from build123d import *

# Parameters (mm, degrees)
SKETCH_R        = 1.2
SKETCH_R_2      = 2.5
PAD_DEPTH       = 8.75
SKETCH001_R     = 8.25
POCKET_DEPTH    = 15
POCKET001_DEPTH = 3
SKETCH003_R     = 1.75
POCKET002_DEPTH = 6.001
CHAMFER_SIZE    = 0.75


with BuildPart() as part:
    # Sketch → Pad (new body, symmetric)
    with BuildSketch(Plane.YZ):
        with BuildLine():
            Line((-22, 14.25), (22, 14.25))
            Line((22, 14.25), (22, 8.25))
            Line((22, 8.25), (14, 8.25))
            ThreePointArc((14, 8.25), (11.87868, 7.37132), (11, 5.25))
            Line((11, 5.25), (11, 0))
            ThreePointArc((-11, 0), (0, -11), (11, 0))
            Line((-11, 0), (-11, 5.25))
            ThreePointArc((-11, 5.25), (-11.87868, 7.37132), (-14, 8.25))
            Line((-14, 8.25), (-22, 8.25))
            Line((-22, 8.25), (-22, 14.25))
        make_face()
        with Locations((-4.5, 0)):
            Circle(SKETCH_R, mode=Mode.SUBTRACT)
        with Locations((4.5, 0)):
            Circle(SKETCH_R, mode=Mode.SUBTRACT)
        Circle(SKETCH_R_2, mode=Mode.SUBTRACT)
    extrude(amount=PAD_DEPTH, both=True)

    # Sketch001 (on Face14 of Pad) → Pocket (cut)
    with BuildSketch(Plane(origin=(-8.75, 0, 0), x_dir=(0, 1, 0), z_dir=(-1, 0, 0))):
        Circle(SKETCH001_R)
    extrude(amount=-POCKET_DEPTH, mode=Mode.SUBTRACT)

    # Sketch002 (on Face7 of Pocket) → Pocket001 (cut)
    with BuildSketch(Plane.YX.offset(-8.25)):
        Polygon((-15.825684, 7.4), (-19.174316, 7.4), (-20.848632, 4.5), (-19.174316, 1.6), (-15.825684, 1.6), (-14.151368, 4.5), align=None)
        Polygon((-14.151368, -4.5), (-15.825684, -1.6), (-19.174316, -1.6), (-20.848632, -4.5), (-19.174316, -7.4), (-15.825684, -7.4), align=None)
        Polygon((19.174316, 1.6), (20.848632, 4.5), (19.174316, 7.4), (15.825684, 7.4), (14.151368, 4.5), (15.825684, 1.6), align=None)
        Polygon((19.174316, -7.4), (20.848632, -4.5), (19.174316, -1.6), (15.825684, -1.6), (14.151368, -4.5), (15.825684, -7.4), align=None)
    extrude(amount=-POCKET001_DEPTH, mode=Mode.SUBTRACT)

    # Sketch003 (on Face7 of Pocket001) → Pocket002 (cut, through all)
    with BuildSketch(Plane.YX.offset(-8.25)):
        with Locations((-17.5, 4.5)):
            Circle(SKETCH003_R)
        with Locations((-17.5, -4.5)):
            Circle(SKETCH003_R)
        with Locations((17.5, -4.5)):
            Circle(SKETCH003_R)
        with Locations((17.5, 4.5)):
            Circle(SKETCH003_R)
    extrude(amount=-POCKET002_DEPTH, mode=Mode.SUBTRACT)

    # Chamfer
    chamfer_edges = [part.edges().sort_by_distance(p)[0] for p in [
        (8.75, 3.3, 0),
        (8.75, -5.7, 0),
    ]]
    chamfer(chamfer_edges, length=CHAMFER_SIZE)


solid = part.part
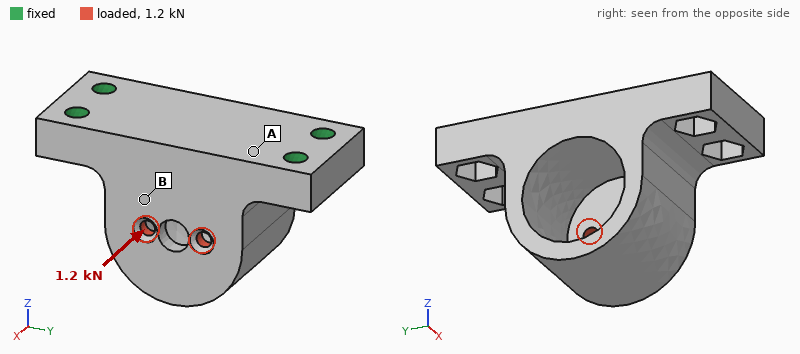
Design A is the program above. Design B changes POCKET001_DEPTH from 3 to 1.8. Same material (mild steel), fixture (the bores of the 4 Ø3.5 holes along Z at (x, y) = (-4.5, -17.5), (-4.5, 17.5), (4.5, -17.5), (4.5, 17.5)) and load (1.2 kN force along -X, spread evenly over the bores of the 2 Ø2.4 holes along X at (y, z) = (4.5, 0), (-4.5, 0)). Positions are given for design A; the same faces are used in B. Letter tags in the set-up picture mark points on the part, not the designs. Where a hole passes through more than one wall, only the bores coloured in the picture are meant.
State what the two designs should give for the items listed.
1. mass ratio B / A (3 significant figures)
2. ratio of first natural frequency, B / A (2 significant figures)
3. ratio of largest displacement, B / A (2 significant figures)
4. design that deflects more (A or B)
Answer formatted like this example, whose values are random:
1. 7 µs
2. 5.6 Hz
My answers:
1. 1.01
2. 1.1
3. 0.91
4. A
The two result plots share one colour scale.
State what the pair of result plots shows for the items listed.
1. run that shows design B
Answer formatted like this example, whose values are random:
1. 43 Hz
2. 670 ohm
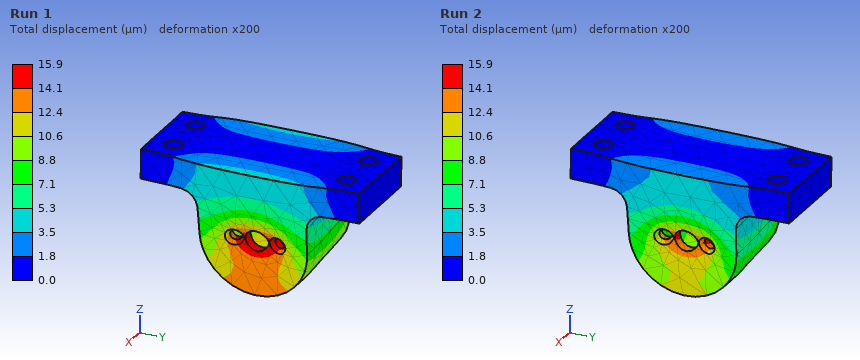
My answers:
1. Run 2
